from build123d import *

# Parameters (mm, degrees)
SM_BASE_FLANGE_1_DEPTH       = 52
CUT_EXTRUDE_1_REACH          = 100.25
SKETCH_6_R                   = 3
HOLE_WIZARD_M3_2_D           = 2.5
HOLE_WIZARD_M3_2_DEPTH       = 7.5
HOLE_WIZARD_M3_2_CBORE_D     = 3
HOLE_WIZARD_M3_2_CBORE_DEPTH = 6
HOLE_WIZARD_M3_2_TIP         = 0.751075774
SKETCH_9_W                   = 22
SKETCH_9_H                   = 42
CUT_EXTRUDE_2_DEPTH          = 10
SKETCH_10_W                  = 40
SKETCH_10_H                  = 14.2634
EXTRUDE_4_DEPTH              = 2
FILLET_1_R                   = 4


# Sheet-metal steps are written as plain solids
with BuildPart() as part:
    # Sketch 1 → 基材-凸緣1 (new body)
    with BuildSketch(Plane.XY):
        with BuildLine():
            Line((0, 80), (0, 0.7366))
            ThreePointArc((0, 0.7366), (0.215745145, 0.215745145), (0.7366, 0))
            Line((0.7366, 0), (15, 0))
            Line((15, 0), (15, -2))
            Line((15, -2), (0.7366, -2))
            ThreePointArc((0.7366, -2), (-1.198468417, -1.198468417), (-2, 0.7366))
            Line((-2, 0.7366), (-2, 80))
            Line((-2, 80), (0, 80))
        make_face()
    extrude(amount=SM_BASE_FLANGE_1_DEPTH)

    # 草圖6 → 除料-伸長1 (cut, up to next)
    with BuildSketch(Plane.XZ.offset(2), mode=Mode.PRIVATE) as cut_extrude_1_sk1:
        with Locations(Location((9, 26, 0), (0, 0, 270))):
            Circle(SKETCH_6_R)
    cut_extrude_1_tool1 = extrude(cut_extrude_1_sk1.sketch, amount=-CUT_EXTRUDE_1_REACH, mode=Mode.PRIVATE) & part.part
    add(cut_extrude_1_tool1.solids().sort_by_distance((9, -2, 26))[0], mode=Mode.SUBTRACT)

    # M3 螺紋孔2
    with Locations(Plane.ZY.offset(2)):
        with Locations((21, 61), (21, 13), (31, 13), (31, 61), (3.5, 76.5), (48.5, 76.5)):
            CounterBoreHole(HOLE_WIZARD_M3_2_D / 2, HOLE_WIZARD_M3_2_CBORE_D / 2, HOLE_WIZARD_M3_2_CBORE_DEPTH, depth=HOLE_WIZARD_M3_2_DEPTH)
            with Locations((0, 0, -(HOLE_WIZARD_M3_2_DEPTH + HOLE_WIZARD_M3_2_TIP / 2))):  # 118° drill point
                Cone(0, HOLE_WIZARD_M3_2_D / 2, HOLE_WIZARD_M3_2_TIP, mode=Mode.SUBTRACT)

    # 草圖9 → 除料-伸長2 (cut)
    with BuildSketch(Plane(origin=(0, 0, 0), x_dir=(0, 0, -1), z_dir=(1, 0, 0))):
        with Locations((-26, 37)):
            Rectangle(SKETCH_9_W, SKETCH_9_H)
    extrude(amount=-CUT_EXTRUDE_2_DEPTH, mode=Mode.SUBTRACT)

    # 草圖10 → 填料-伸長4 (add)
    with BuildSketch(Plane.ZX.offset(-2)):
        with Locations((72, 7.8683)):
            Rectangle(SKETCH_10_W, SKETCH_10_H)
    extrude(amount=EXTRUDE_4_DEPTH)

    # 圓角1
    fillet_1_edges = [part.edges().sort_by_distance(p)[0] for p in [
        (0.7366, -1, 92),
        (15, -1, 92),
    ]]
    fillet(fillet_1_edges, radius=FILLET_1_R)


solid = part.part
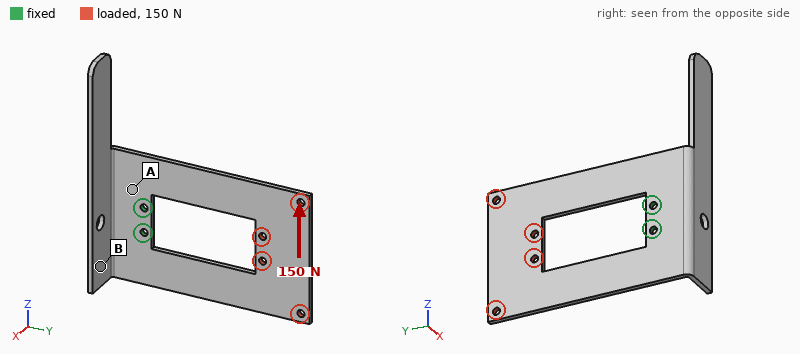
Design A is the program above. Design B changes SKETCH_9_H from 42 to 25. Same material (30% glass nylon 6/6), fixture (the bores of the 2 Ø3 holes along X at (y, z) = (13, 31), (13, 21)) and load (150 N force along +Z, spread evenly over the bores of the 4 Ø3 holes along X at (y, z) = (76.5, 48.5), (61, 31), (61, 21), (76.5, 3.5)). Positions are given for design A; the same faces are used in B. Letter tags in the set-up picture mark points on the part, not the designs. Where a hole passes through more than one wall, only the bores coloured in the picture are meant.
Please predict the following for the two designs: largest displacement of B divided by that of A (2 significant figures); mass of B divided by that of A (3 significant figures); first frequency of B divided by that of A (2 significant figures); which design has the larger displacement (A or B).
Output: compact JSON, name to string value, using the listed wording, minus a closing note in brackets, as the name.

{"largest displacement of B divided by that of A": "0.54", "mass of B divided by that of A": "1.08", "first frequency of B divided by that of A": "1.2", "which design has the larger displacement": "A"}
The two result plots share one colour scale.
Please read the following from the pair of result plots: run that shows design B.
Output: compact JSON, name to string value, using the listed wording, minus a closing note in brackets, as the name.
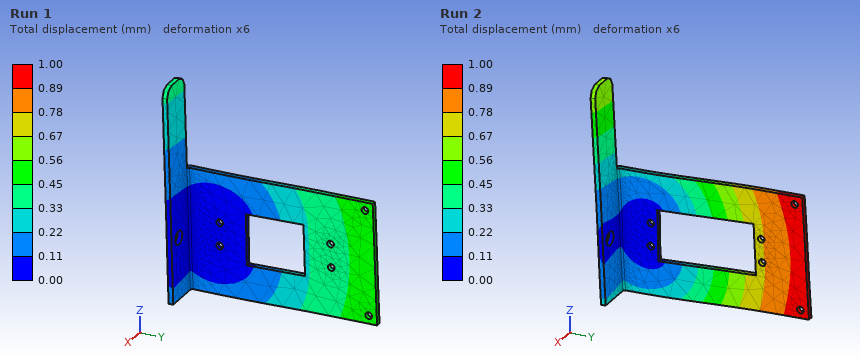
{"run that shows design B": "Run 1"}
